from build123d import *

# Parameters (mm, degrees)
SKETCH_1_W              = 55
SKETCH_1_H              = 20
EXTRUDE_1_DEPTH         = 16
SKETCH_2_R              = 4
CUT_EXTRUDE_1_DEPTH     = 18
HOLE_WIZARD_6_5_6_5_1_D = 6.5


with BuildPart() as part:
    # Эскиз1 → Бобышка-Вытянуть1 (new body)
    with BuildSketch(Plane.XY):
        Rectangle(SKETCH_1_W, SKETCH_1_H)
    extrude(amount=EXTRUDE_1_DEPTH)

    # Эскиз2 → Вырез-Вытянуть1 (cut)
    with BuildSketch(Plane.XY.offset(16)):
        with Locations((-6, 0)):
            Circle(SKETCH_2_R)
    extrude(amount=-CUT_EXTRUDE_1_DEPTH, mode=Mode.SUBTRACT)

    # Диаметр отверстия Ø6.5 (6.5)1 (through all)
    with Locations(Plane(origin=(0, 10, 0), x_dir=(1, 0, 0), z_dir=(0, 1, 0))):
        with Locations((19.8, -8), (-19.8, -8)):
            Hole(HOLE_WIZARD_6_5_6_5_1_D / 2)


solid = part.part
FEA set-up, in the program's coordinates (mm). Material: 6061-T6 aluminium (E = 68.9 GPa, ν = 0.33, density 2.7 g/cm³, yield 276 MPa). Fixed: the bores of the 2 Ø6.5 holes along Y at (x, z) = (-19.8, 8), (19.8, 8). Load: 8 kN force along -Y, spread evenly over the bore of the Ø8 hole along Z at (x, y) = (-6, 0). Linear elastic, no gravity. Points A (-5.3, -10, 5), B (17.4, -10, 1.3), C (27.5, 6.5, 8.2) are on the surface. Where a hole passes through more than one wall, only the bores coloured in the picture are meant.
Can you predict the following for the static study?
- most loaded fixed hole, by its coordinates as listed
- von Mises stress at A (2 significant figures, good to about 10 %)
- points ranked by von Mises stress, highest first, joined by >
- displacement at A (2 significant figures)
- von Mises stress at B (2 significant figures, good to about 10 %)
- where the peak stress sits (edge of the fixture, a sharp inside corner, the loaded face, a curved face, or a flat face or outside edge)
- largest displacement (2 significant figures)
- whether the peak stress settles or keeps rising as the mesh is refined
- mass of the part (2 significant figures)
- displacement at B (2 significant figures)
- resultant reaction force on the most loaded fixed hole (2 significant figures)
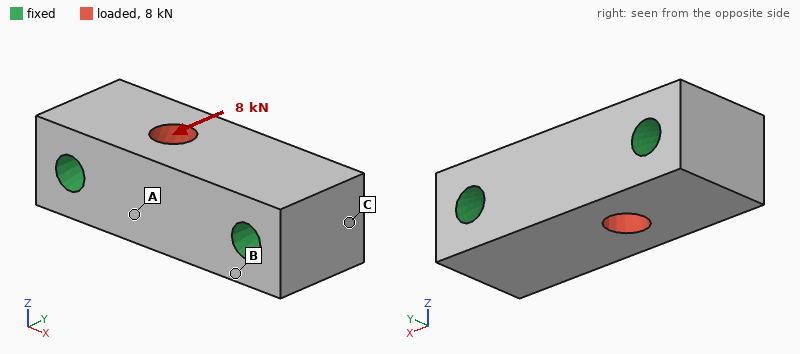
(-19.8, 8)
37 MPa
A > B > C
10 µm
16 MPa
edge of the fixture
13 µm
keeps rising
42 g
2.0 µm
5.3 kN
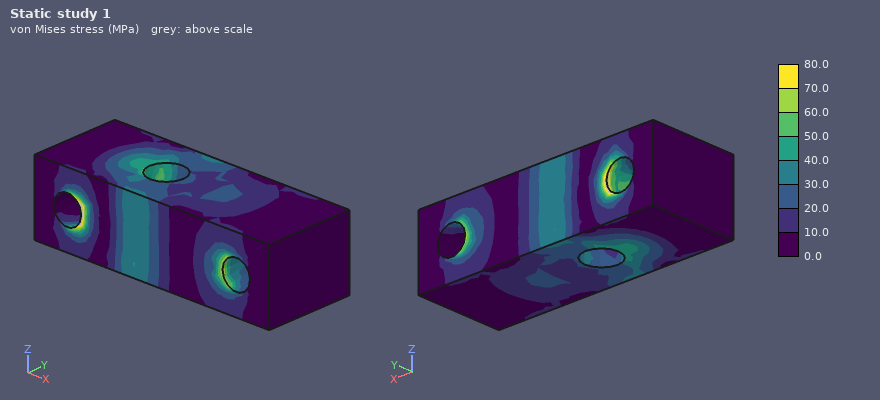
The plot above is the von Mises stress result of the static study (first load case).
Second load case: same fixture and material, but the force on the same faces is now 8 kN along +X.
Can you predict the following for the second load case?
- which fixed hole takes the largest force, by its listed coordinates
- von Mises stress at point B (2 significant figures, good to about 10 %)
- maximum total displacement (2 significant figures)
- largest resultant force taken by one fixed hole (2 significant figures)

(-19.8, 8)
5.3 MPa
4.1 µm
5.0 kN
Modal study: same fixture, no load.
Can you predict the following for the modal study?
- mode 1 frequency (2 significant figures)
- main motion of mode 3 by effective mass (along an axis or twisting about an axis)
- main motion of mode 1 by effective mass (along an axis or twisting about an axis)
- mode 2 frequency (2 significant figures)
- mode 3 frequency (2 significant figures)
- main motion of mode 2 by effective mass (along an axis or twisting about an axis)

29 kHz
twisting about X
along Z
34 kHz
38 kHz
along Y
